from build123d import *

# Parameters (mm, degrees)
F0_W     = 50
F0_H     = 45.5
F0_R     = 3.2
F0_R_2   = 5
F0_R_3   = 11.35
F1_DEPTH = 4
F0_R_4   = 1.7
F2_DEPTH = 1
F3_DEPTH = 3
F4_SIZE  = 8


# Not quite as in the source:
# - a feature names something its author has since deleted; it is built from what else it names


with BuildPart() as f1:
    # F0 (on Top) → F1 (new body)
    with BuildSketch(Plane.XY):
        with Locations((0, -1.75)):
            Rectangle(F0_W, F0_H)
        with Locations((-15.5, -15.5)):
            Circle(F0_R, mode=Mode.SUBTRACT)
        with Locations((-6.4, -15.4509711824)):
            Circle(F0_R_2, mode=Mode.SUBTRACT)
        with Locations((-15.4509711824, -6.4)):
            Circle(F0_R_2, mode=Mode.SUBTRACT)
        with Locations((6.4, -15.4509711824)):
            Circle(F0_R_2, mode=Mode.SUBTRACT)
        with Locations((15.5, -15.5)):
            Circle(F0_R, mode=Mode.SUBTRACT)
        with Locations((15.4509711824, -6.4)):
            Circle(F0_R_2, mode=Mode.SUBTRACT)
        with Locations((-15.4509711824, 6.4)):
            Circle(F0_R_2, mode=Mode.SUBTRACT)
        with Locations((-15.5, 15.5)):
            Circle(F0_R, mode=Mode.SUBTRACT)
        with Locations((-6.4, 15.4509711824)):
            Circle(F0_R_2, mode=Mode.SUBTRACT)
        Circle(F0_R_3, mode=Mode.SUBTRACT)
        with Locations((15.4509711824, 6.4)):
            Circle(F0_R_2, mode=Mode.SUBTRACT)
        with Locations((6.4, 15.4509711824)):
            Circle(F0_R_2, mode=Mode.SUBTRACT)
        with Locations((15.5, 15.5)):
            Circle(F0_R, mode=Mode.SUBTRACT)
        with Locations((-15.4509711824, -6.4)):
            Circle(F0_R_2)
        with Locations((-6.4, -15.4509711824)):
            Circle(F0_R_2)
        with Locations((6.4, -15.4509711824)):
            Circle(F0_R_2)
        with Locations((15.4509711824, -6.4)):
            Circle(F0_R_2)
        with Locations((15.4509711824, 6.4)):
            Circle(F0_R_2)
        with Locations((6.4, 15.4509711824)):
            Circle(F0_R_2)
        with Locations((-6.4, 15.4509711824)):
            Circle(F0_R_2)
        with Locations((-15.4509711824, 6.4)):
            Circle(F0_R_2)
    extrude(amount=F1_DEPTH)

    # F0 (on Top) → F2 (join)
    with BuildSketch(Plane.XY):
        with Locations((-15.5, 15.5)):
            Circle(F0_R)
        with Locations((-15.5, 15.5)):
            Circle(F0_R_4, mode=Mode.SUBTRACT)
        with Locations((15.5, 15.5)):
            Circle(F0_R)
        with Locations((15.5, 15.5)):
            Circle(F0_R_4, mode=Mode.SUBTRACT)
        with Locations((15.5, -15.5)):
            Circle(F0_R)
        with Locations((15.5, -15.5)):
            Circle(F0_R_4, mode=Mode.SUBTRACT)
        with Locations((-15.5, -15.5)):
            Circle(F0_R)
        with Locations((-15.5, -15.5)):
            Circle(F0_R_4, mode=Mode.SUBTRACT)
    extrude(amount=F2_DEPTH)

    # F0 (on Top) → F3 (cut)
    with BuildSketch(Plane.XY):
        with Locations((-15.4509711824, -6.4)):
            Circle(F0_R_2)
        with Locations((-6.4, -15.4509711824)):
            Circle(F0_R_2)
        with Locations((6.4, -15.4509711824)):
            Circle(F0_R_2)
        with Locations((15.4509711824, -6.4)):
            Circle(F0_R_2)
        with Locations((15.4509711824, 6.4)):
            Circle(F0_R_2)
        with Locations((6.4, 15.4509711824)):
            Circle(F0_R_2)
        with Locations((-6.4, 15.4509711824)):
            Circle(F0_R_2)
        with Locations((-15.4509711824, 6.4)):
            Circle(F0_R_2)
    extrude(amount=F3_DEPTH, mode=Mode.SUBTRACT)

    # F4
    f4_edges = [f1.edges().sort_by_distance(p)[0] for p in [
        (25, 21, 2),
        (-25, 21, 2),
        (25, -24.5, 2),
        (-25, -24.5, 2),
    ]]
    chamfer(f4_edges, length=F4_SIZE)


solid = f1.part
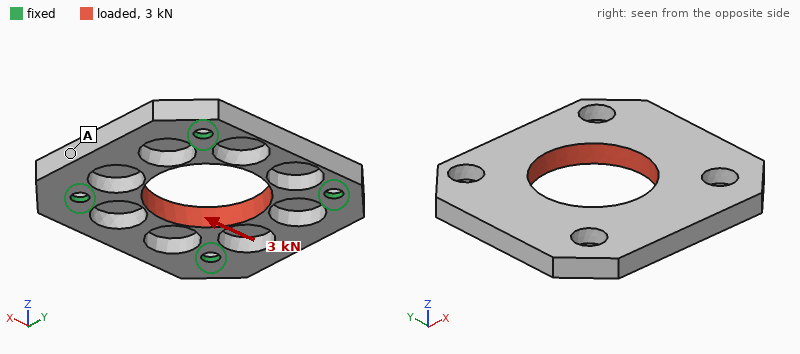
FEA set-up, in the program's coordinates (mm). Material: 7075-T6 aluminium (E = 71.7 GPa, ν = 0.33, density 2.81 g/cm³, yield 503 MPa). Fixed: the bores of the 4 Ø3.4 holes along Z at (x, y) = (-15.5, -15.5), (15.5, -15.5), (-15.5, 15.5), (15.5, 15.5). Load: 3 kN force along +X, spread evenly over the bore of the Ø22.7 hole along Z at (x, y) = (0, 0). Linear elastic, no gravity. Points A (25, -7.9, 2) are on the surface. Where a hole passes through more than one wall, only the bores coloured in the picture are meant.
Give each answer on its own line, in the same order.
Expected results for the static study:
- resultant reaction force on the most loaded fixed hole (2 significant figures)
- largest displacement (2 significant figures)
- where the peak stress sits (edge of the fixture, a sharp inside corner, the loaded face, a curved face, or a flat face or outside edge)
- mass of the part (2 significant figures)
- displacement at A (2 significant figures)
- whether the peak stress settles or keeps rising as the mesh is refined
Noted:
770 N
28 µm
edge of the fixture
13 g
23 µm
keeps rising
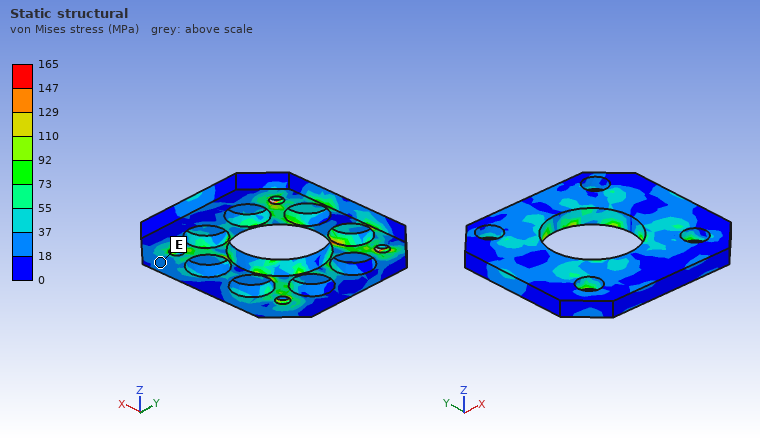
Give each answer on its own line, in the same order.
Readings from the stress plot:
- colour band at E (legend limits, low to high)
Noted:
18 to 37 MPa
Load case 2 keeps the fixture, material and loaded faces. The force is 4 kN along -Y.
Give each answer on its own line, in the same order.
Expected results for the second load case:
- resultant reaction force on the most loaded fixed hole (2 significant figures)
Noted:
1.0 kN
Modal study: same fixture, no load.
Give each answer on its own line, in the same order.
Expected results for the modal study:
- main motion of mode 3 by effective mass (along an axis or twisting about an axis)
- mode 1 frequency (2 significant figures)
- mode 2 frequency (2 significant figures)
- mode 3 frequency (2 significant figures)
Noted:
along Z
9900 Hz
11 kHz
13 kHz
